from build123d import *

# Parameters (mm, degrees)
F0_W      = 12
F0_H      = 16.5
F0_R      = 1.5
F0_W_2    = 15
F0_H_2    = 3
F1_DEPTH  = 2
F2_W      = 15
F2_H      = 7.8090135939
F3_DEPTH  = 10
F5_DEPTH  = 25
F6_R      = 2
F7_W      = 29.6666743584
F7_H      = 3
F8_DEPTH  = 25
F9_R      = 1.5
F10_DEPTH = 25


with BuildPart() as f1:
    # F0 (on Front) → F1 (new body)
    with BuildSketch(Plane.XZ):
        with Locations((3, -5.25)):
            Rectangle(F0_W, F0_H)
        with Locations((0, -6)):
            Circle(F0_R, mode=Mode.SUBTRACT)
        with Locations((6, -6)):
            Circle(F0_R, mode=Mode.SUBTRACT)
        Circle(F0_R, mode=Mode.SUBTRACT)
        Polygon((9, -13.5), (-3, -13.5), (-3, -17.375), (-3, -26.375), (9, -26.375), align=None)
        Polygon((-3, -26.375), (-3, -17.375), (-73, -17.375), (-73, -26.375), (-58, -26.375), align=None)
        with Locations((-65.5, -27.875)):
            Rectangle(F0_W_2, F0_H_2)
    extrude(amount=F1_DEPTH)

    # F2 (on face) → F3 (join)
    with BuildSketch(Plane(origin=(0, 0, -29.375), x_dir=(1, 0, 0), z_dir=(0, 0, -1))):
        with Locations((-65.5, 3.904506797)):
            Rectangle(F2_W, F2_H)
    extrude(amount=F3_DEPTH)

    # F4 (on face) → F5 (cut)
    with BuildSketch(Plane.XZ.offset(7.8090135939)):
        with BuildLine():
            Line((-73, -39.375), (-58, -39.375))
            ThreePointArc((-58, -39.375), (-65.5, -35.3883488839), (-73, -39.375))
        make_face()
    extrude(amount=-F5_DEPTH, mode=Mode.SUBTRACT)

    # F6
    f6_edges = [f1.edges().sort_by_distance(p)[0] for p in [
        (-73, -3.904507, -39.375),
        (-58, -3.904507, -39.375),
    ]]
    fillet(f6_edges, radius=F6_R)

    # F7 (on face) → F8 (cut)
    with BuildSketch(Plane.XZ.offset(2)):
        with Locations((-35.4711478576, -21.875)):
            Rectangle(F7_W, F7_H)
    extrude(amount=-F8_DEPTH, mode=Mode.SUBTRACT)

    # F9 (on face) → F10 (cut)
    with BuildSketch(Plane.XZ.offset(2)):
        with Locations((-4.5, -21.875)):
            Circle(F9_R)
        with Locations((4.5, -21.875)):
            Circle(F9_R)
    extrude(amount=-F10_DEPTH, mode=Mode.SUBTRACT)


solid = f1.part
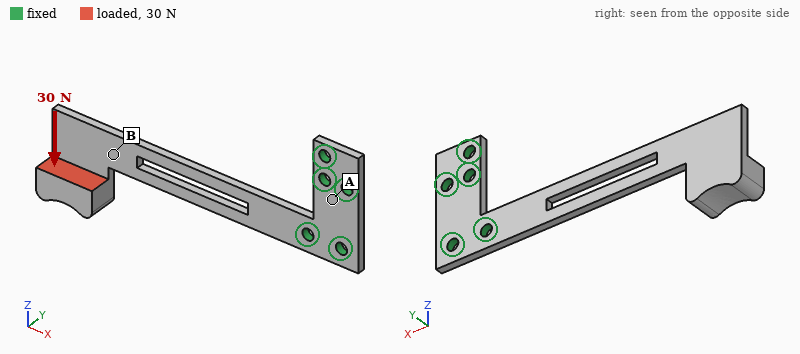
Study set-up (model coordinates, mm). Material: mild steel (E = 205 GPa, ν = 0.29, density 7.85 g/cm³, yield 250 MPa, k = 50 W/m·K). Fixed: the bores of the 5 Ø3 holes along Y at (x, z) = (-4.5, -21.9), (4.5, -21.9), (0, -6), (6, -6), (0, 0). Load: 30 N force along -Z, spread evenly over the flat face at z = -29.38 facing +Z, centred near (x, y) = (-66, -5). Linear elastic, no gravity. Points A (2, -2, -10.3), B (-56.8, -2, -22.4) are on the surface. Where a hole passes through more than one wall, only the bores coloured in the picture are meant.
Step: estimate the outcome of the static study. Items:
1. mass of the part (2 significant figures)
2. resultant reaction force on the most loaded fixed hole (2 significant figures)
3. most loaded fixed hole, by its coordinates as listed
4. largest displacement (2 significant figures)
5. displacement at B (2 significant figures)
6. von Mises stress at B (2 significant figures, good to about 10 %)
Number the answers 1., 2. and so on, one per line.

1. 20 g
2. 110 N
3. (-4.5, -21.9)
4. 0.23 mm
5. 0.13 mm
6. 23 MPa
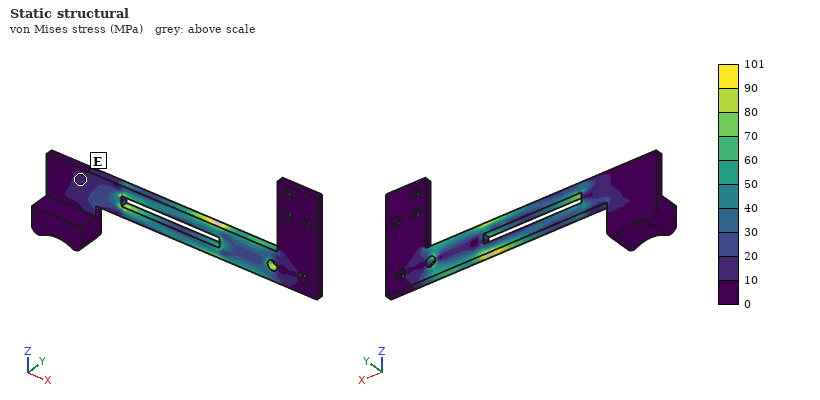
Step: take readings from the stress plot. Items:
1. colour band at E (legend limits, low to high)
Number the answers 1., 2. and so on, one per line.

1. 10 to 20 MPa
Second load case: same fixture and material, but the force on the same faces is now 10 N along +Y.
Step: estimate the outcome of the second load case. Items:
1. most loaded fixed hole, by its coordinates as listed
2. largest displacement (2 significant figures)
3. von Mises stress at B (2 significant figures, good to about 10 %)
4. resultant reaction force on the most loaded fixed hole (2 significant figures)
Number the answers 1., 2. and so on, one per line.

1. (-4.5, -21.9)
2. 0.92 mm
3. 18 MPa
4. 18 N
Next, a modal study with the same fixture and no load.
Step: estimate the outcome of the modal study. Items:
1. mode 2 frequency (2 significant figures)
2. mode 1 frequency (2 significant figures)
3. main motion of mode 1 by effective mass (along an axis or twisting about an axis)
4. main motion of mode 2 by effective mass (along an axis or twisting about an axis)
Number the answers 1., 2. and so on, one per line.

1. 680 Hz
2. 180 Hz
3. along Y
4. along Z
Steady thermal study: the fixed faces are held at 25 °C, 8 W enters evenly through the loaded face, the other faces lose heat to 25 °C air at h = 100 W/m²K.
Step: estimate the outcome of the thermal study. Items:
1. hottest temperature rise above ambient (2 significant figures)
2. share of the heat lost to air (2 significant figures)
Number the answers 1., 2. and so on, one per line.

1. 85 K
2. 97 %
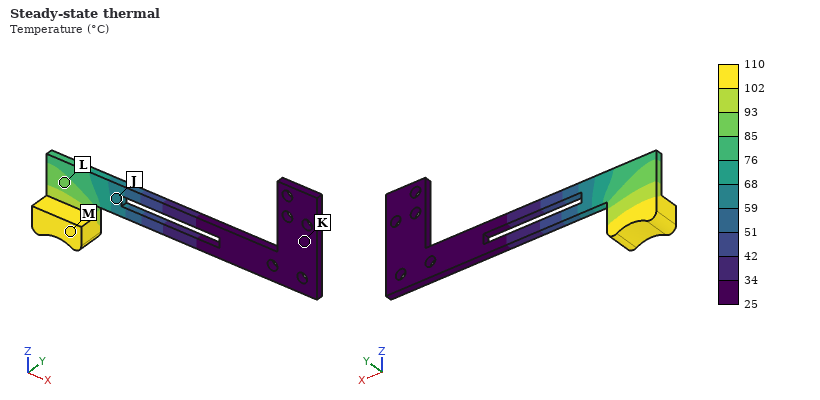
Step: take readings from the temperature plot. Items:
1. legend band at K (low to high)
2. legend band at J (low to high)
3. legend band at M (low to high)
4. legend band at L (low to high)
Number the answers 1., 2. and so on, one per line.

1. 25 to 34 °C
2. 59 to 68 °C
3. 102 to 110 °C
4. 85 to 93 °C
